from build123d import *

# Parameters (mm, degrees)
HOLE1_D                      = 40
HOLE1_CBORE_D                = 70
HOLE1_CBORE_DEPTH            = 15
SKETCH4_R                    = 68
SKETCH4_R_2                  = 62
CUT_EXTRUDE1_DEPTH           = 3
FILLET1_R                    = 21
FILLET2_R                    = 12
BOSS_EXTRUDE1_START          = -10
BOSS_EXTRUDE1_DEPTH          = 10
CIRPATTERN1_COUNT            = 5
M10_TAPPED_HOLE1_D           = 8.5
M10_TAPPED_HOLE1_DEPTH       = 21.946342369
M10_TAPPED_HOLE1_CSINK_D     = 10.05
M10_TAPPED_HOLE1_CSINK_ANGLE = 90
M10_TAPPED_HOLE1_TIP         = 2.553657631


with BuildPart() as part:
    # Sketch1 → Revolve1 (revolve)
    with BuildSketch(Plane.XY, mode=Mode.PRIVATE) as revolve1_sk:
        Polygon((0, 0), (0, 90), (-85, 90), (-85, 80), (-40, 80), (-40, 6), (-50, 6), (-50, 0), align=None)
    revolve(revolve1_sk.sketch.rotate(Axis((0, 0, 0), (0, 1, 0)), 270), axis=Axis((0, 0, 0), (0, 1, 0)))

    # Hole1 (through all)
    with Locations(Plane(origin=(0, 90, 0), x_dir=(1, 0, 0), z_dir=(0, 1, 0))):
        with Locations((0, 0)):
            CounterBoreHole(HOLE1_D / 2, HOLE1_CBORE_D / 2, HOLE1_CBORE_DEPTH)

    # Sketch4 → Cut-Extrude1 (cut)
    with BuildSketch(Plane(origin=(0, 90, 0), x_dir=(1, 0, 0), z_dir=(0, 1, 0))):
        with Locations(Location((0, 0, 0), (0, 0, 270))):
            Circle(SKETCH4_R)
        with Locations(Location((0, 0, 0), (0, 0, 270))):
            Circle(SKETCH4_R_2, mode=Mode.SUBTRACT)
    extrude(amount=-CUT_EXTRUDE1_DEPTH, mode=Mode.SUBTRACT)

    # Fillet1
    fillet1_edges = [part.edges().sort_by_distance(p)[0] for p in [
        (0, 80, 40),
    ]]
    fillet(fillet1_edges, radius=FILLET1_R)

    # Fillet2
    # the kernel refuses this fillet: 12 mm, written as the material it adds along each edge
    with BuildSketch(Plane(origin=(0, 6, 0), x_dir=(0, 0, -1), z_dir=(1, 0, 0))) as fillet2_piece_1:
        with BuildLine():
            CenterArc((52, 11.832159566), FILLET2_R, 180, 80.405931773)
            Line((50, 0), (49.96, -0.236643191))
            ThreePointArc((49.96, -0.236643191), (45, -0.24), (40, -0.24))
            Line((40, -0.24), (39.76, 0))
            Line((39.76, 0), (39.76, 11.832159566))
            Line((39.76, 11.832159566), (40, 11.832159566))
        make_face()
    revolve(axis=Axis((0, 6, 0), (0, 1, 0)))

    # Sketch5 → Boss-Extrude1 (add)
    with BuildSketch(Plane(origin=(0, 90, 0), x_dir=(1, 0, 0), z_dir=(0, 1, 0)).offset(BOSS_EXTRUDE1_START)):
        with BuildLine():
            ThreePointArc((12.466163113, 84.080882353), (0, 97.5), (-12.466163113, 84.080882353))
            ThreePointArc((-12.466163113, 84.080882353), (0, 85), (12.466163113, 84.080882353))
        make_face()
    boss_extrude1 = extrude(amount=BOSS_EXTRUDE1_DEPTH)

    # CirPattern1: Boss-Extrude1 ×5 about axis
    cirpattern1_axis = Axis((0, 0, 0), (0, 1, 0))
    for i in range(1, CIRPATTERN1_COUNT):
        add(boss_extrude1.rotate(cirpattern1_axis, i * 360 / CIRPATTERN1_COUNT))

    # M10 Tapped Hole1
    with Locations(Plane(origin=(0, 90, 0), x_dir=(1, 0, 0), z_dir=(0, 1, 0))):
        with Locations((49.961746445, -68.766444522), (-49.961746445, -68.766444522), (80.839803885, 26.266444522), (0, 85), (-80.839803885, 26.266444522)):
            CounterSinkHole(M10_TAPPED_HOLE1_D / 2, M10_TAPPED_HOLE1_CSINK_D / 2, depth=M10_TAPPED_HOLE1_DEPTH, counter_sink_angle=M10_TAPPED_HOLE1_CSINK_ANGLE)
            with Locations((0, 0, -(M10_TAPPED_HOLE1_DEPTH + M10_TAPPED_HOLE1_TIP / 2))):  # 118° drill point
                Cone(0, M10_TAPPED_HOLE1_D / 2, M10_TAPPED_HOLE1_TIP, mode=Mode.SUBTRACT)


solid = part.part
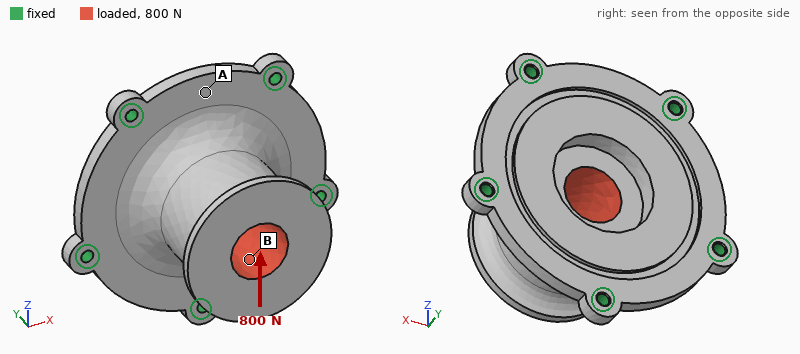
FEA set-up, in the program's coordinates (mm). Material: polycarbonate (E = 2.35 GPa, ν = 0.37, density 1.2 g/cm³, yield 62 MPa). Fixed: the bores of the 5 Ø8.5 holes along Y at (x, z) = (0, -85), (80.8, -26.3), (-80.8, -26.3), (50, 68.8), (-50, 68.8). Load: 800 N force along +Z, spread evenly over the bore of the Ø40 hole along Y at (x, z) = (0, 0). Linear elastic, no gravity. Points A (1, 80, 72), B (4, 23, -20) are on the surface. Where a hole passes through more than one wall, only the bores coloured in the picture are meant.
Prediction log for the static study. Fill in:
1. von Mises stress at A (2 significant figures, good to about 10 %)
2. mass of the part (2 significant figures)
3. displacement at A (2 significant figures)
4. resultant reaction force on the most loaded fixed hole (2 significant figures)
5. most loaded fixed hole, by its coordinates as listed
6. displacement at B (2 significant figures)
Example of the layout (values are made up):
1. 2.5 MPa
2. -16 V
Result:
1. 1.2 MPa
2. 640 g
3. 0.088 mm
4. 340 N
5. (0, -85)
6. 0.16 mm
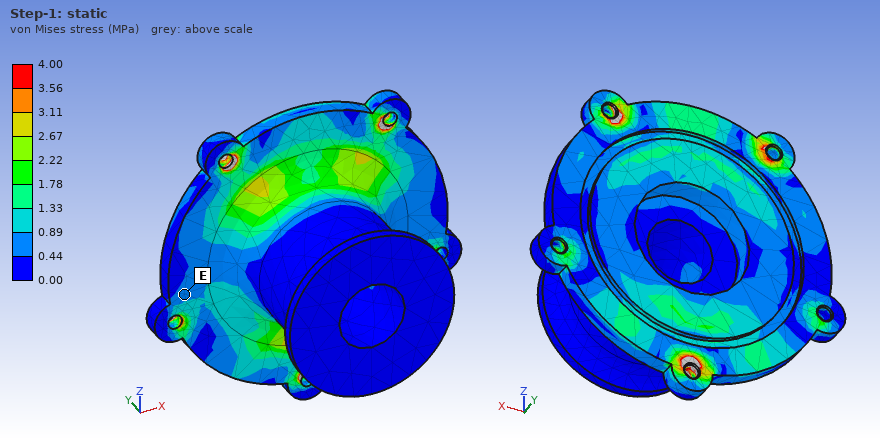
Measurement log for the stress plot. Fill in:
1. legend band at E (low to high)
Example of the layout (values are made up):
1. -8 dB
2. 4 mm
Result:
1. 0.44 to 0.89 MPa
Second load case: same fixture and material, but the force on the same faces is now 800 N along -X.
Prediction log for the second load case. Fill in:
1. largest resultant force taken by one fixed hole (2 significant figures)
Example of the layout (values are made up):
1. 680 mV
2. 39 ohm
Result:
1. 320 N
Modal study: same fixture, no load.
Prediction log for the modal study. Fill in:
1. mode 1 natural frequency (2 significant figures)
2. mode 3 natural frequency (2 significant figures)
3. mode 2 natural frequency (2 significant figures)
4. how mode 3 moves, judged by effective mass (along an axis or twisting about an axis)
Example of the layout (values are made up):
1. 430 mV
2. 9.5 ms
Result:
1. 520 Hz
2. 580 Hz
3. 520 Hz
4. along Y
